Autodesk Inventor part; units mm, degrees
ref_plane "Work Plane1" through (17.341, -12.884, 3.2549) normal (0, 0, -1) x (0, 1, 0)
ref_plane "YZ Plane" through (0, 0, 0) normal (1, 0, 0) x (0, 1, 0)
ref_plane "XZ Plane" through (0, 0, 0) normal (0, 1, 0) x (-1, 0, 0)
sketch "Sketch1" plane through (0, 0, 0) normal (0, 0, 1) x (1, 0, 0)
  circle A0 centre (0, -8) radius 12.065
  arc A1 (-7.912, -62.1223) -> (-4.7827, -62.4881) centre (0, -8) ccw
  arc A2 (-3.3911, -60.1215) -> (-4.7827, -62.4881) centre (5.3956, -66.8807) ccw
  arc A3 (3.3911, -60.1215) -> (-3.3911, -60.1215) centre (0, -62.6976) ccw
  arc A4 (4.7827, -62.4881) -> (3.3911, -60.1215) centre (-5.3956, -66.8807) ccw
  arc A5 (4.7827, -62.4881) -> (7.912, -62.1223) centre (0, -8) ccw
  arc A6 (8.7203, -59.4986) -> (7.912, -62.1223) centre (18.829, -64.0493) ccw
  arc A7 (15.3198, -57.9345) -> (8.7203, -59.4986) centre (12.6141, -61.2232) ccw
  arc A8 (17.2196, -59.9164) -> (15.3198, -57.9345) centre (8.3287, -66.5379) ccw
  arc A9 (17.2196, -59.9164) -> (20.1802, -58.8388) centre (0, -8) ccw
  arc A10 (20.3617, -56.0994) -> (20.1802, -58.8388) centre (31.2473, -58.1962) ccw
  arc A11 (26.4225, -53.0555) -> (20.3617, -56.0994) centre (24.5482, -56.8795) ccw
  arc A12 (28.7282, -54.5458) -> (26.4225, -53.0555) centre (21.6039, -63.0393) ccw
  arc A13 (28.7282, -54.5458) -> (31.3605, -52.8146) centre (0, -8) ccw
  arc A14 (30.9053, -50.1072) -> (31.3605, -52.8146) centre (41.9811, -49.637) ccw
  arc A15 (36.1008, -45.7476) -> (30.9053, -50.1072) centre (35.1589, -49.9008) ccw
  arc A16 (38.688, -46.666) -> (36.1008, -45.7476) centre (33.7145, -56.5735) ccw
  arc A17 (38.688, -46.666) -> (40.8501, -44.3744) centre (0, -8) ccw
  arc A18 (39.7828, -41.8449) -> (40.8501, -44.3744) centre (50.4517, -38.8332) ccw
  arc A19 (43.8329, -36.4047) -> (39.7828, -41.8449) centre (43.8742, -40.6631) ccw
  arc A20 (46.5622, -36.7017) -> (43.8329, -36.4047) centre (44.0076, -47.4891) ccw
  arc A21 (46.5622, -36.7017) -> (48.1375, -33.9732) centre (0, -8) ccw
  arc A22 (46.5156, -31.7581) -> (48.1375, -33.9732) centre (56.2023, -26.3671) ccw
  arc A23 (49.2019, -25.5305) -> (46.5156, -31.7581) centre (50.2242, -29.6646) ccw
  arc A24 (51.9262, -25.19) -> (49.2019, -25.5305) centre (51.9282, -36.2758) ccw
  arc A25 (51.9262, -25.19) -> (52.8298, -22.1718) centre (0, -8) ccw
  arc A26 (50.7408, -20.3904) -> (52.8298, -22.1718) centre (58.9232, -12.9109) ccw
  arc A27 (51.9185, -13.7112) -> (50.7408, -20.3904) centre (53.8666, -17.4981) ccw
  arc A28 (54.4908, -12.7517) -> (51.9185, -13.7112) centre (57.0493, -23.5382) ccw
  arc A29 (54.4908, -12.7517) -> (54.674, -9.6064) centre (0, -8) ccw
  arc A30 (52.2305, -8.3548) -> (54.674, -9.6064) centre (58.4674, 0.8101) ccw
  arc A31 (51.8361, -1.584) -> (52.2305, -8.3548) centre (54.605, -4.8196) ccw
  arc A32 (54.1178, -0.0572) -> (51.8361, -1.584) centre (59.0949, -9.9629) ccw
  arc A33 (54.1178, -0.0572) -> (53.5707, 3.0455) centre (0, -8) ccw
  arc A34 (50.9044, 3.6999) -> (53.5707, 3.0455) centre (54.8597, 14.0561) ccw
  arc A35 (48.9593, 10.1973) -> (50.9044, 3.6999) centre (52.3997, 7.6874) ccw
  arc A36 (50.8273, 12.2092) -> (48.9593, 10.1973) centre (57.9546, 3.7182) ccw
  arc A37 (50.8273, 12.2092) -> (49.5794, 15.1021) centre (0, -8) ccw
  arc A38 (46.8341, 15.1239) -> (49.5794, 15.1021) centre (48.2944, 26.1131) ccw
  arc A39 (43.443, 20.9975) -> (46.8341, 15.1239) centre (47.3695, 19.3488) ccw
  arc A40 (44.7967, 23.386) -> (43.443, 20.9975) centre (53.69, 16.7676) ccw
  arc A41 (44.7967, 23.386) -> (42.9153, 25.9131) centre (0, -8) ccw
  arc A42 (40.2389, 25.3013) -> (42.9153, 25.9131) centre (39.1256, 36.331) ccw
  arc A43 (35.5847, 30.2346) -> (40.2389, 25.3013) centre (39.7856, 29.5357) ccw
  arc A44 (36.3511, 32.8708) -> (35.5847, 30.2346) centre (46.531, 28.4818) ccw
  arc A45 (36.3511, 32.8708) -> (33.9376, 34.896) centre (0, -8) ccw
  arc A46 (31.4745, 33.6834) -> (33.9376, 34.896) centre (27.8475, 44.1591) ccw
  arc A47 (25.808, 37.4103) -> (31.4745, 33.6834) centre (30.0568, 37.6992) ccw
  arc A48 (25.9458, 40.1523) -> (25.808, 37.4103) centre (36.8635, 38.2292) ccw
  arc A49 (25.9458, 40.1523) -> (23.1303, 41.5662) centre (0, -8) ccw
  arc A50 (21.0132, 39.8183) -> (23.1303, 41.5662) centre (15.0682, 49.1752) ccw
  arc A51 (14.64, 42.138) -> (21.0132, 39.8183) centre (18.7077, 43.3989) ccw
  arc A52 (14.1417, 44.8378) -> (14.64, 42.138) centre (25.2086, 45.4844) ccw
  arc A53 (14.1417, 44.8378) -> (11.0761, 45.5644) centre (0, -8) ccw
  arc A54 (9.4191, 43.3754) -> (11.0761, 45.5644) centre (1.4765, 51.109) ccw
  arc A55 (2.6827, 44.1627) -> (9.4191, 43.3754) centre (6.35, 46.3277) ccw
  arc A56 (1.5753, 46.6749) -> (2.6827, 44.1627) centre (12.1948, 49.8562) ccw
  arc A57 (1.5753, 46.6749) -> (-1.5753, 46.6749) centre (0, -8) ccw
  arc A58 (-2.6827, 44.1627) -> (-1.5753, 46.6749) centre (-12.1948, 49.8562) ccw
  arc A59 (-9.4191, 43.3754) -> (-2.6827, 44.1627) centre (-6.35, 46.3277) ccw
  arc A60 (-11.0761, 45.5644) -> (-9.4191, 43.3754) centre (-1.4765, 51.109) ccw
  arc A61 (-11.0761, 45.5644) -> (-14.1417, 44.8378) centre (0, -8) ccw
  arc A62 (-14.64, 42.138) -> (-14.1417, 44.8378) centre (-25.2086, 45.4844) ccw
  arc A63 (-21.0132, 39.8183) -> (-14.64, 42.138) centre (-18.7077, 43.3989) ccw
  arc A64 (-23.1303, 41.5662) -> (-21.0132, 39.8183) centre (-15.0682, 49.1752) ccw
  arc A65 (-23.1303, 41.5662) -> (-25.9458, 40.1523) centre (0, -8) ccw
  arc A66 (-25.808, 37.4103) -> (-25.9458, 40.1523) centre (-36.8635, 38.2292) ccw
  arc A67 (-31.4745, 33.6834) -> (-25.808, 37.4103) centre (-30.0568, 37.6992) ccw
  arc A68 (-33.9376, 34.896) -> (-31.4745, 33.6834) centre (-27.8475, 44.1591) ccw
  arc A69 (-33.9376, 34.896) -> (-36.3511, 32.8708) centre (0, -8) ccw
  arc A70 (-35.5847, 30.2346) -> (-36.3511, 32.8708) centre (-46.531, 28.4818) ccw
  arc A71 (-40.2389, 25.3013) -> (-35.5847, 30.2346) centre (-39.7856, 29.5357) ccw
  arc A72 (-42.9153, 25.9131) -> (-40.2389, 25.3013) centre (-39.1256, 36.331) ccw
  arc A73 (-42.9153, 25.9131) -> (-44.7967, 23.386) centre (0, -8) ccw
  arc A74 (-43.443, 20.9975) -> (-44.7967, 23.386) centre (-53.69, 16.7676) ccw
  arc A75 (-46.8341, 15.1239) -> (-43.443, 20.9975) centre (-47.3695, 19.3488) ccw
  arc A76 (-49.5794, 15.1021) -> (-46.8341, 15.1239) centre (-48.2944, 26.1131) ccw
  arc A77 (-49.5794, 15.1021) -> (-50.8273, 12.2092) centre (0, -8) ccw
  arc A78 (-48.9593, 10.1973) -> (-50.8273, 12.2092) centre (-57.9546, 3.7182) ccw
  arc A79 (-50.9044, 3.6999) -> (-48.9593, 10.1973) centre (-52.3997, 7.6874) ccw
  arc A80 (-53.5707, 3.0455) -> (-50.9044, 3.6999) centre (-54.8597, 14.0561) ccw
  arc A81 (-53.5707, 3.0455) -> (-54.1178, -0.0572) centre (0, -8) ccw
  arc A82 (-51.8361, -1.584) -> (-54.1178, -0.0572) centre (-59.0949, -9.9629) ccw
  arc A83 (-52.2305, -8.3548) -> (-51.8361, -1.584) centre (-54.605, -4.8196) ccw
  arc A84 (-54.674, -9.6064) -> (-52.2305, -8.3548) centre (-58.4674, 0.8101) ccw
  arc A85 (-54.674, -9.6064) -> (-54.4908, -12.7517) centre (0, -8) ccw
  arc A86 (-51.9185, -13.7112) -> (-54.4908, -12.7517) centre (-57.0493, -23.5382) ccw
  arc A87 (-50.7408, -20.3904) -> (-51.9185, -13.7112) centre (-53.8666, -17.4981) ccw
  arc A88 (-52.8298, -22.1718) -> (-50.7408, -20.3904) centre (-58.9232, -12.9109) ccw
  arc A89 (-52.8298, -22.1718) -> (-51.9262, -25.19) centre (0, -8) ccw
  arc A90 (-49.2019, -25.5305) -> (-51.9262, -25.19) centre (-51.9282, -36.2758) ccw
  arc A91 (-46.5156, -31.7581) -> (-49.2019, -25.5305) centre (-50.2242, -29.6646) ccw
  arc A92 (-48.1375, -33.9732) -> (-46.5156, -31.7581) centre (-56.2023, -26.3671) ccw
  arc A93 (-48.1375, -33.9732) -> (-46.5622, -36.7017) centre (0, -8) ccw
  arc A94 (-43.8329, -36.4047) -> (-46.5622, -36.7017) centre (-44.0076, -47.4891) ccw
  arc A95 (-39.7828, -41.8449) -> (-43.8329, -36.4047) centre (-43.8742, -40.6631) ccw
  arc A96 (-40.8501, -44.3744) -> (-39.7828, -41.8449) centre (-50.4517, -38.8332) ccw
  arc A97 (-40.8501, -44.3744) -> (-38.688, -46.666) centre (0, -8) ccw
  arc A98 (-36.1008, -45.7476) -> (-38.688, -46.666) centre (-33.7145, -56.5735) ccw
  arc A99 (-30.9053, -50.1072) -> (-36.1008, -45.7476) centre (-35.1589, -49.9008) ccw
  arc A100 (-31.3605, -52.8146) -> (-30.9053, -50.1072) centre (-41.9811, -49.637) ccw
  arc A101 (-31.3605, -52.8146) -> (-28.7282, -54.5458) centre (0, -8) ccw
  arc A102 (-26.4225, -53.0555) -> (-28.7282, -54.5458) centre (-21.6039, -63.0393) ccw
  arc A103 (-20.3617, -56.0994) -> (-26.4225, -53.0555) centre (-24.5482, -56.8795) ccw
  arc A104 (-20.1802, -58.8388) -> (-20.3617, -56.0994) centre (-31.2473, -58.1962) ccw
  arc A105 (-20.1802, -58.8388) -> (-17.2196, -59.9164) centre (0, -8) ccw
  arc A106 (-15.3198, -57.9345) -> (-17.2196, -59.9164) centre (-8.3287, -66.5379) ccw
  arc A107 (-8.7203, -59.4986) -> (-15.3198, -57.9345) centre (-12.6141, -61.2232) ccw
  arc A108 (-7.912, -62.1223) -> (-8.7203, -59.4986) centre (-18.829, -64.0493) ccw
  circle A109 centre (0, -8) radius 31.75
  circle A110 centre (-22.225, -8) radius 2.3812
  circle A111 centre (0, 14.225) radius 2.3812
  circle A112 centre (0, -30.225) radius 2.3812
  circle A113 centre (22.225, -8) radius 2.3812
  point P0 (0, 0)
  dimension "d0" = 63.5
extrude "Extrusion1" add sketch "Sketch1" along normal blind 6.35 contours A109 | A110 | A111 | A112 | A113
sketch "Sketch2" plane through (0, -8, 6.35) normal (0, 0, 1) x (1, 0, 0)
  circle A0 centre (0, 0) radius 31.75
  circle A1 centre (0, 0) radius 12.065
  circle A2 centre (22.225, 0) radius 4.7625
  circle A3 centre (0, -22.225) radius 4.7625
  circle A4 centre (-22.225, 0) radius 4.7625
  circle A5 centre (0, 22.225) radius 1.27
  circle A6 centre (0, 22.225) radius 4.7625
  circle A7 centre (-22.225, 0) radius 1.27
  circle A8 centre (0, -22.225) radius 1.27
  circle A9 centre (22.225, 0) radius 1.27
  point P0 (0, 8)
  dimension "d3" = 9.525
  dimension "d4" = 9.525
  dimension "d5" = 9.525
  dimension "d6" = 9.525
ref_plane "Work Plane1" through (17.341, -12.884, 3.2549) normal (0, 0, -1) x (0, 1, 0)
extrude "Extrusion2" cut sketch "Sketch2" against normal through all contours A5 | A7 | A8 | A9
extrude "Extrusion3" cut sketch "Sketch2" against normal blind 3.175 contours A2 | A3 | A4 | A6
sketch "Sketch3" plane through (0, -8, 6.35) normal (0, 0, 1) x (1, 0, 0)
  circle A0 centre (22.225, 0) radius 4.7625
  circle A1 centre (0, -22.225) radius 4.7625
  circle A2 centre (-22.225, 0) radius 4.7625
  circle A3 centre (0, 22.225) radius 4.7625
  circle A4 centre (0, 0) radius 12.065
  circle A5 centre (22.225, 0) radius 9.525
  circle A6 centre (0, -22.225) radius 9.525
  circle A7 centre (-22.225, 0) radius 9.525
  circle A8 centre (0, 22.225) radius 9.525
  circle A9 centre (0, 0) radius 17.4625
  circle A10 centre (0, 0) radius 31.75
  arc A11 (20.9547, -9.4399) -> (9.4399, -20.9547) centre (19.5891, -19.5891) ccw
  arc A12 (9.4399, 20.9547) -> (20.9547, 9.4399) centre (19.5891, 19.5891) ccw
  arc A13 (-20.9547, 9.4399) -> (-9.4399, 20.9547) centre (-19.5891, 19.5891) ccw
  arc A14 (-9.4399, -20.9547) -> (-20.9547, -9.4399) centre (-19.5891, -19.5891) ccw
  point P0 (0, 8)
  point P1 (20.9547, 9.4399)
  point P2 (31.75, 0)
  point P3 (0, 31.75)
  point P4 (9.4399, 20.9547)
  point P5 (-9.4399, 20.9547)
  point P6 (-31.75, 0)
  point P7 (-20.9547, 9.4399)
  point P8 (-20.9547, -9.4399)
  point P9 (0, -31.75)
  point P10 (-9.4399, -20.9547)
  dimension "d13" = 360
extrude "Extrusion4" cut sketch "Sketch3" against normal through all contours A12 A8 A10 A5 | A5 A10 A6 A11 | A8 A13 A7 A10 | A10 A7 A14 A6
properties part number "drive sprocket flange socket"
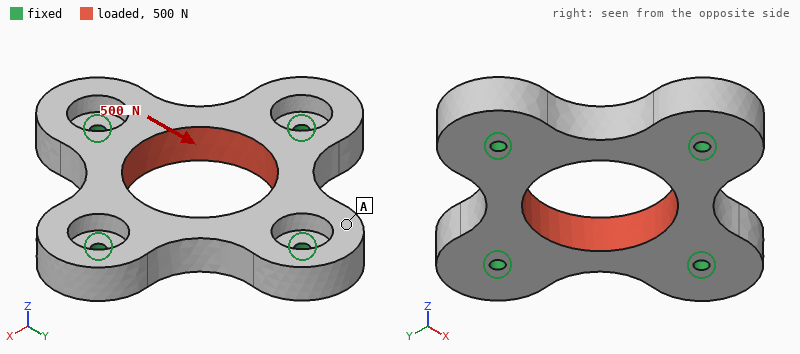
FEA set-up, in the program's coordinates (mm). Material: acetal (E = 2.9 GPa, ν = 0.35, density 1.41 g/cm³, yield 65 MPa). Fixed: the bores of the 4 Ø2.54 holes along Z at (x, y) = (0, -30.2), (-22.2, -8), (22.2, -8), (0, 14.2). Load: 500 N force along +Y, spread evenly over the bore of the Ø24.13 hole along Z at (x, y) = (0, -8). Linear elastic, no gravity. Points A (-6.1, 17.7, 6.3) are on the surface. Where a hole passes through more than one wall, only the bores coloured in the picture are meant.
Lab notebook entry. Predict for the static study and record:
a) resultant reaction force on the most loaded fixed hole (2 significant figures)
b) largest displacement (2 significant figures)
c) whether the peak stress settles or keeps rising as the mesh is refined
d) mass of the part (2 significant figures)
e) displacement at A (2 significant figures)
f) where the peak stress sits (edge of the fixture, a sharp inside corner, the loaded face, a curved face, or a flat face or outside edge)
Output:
170 N
29 µm
keeps rising
12 g
17 µm
edge of the fixture
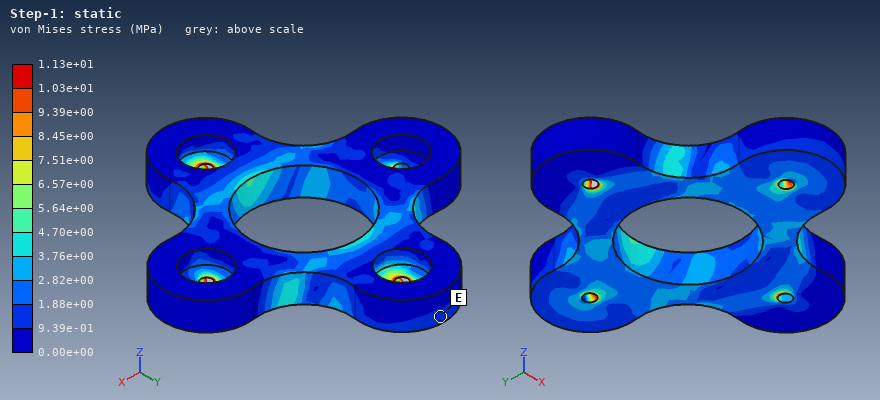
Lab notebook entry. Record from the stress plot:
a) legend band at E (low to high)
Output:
9.39e-01 to 1.88e+00 MPa
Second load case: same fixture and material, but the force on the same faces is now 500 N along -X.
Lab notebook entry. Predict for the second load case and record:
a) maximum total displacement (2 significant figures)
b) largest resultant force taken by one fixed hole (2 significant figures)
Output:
29 µm
170 N
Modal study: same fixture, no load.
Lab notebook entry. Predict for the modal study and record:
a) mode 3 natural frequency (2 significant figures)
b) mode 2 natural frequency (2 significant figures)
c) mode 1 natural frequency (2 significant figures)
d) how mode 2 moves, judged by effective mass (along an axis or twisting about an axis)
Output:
5300 Hz
4900 Hz
4500 Hz
along Z
